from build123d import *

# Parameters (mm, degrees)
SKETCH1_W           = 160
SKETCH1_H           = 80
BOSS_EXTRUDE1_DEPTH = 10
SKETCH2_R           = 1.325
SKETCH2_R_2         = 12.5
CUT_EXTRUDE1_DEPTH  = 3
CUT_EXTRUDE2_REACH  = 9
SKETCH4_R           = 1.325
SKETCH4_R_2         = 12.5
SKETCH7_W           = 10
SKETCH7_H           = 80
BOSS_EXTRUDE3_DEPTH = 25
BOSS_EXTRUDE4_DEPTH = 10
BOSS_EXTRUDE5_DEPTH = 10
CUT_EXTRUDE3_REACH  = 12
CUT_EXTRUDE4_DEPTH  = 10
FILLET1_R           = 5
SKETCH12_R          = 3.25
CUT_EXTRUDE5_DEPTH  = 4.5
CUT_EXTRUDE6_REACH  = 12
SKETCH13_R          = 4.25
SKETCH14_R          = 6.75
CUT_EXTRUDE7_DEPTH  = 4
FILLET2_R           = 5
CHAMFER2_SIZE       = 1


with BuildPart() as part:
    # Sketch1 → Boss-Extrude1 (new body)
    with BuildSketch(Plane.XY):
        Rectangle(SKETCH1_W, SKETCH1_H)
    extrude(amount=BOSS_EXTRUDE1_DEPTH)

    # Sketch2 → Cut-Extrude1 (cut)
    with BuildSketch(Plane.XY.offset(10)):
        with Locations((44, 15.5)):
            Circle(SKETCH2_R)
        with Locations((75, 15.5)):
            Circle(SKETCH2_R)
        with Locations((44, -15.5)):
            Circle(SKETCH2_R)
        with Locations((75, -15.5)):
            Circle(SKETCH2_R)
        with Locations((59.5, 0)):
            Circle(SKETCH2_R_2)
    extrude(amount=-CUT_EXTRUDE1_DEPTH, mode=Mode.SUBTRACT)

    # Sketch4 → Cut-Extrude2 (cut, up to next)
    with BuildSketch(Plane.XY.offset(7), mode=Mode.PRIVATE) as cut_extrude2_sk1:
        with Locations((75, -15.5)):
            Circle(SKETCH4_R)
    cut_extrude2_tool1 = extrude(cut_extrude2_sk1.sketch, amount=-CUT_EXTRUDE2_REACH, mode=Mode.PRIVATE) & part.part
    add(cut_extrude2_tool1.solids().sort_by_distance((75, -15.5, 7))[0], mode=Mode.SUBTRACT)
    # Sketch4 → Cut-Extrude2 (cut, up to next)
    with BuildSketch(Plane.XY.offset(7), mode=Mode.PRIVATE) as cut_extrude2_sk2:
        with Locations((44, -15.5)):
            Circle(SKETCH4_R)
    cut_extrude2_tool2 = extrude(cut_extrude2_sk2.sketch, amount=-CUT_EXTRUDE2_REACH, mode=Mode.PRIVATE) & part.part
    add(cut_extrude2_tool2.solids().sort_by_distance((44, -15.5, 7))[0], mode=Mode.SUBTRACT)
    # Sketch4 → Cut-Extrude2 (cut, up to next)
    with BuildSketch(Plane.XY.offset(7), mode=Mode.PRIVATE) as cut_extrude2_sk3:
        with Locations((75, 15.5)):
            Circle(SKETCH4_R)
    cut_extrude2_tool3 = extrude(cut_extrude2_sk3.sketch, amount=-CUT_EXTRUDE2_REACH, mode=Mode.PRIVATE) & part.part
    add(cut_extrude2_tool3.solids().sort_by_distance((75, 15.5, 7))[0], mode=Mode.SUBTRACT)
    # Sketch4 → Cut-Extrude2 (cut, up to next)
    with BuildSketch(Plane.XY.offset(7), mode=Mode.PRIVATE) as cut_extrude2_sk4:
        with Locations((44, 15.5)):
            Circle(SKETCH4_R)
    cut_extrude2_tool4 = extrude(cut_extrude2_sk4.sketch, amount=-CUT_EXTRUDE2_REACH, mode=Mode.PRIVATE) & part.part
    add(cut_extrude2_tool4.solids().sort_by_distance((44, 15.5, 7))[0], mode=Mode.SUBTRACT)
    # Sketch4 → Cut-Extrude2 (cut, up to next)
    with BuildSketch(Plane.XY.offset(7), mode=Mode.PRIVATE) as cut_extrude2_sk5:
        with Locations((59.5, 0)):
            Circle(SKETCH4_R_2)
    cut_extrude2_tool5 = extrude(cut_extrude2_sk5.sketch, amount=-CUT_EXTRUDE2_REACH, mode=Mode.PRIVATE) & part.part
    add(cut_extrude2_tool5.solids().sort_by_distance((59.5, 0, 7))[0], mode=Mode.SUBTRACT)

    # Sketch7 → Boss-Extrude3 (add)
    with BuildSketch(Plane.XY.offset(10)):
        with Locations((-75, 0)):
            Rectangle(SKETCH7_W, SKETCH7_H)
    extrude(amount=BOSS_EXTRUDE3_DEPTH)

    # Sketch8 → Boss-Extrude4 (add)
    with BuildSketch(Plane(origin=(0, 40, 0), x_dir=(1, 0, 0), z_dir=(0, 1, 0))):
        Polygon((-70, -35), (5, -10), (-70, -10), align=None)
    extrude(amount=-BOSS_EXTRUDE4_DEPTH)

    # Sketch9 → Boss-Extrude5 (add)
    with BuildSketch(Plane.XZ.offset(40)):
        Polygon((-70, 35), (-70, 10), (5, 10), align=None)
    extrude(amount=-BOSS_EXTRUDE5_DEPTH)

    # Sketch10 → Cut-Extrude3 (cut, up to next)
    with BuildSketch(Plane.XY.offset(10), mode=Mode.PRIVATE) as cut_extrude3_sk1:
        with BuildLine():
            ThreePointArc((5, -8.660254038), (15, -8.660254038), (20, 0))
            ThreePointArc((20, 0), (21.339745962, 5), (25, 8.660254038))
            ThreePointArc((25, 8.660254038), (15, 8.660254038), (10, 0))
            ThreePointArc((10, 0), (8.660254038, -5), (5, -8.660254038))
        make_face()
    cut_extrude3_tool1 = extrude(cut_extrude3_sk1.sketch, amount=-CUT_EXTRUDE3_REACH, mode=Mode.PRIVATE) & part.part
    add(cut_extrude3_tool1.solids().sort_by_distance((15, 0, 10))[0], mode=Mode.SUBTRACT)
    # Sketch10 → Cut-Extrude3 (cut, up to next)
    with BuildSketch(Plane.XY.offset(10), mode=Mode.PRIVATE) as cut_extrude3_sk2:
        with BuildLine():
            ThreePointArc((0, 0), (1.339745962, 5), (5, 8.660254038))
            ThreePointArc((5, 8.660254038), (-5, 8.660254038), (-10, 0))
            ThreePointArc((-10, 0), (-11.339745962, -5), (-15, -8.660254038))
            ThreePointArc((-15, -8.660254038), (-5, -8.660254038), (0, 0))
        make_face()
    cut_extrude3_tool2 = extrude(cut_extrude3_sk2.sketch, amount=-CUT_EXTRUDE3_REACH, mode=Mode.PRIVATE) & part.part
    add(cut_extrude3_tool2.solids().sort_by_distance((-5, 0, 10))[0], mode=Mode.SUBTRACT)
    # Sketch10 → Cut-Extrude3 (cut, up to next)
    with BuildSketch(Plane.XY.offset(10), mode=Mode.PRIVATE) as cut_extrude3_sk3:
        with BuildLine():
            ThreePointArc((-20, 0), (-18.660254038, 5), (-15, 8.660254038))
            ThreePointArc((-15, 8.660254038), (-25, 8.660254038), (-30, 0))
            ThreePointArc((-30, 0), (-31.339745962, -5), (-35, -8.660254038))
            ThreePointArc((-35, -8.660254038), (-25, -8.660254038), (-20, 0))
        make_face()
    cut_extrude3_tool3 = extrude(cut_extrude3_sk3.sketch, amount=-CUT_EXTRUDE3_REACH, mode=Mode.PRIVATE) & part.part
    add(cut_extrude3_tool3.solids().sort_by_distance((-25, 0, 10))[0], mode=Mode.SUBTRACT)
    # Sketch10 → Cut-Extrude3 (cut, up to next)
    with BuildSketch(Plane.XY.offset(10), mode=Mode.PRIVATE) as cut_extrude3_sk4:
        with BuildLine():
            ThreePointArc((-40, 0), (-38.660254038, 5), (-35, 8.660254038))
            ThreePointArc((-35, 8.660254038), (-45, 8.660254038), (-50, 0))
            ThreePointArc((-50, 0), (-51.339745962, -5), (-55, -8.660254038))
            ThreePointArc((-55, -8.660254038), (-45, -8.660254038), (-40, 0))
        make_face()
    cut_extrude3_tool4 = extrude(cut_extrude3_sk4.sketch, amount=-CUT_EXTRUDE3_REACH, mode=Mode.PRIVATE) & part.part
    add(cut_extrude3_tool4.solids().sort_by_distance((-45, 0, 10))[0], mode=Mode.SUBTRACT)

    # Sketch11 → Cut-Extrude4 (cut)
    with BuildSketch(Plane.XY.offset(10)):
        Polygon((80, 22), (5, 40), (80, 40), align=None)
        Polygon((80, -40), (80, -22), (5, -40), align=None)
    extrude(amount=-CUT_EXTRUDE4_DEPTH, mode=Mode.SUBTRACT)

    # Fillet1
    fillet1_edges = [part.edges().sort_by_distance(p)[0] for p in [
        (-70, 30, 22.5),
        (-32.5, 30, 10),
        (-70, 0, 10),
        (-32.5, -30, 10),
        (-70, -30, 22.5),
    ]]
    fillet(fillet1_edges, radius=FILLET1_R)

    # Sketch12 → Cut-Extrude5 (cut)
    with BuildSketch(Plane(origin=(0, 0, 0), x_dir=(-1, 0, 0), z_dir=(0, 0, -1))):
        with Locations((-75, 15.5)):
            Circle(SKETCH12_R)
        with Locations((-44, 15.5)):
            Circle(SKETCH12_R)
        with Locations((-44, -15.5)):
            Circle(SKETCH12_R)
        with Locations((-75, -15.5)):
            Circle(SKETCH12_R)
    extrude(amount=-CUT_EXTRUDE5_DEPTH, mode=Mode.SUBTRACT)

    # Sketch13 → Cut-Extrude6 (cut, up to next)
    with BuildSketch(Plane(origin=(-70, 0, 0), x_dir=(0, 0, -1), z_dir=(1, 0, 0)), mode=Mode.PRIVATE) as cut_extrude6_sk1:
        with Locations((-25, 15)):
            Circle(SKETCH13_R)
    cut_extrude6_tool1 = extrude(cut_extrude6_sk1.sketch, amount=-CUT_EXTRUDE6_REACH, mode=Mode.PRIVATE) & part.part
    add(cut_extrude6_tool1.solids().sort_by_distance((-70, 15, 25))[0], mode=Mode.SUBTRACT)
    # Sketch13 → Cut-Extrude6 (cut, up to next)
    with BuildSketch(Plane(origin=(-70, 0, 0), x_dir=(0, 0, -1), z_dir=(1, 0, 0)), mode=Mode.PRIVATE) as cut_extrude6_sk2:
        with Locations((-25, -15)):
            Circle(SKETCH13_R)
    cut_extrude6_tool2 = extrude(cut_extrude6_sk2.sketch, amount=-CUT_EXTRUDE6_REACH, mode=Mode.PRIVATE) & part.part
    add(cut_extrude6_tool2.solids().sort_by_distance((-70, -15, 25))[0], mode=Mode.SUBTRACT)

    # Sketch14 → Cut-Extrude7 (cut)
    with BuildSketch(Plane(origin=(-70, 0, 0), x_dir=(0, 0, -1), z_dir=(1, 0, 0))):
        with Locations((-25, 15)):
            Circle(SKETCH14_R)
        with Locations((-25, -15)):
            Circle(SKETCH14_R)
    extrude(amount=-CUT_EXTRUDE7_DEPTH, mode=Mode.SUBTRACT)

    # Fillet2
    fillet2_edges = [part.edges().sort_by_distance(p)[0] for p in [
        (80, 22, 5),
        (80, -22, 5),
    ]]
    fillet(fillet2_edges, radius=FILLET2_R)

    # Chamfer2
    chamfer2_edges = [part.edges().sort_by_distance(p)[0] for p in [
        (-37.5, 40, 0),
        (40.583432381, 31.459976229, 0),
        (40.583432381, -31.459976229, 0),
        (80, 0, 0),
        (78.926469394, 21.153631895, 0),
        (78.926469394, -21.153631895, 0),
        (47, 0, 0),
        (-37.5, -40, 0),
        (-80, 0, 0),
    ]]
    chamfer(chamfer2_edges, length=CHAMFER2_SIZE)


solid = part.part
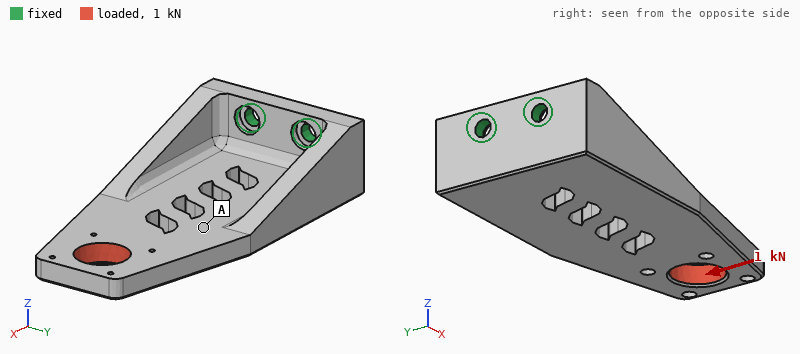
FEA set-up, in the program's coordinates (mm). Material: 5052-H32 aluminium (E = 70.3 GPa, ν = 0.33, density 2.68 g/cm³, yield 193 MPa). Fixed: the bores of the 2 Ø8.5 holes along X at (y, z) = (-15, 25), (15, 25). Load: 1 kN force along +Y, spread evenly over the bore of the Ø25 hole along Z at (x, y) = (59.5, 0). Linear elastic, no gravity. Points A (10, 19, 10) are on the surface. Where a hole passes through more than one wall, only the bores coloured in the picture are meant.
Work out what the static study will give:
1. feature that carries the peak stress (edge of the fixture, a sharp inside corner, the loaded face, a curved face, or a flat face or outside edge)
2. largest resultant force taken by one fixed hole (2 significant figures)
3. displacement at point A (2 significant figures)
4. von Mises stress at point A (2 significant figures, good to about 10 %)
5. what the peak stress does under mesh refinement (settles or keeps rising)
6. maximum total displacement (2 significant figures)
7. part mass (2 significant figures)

edge of the fixture
3.6 kN
0.15 mm
9.7 MPa
keeps rising
0.28 mm
370 g
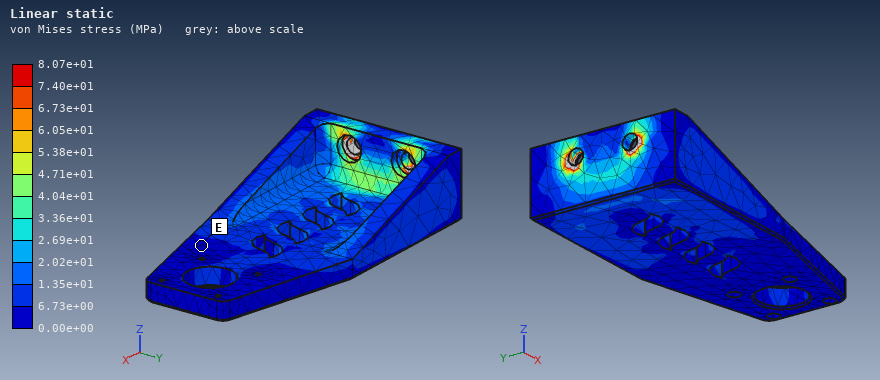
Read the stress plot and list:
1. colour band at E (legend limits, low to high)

0.00e+00 to 6.73e+00 MPa
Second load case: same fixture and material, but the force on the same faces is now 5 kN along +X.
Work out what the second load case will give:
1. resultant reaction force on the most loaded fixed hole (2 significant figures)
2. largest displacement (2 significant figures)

2.5 kN
0.51 mm
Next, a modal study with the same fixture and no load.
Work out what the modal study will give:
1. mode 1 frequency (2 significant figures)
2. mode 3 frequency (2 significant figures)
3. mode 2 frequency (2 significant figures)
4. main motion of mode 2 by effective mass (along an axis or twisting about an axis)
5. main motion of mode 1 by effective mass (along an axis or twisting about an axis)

500 Hz
2000 Hz
1000 Hz
along Y
along Z
